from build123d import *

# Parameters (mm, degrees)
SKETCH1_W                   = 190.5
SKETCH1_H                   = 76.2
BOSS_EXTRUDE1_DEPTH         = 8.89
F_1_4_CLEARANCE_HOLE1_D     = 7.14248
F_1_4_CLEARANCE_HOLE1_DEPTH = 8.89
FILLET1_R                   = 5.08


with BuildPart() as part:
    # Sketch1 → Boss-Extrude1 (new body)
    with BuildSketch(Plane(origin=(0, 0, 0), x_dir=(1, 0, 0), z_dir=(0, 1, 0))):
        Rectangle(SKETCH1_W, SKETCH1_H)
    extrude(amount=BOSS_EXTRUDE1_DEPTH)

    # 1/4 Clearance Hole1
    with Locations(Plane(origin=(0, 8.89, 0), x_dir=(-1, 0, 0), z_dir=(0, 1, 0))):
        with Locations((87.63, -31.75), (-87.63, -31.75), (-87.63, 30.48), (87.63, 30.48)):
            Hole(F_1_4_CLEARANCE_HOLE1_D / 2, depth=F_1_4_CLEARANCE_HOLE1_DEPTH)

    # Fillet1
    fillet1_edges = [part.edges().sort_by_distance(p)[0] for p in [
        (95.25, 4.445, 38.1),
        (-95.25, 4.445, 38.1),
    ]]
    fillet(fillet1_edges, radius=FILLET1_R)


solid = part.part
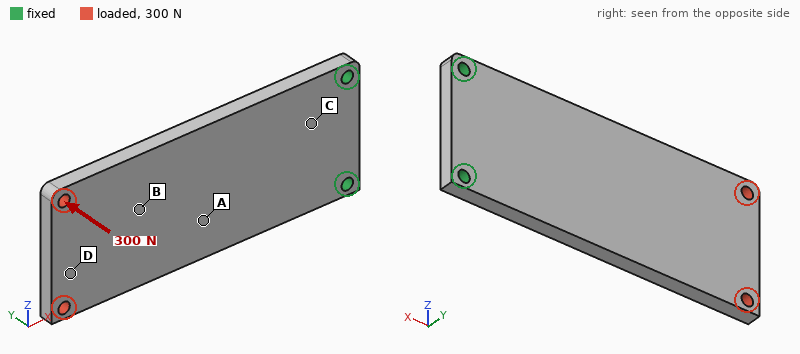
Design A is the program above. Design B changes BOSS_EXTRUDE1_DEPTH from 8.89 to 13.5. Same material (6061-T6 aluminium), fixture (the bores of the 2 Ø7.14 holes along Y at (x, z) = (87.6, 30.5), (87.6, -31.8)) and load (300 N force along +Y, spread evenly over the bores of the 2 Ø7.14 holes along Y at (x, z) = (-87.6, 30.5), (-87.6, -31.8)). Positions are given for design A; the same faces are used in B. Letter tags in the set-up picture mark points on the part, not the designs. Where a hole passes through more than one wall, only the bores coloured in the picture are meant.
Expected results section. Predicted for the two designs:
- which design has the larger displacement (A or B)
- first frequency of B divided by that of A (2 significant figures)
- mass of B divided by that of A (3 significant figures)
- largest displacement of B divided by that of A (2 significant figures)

A
1.5
1.52
0.30
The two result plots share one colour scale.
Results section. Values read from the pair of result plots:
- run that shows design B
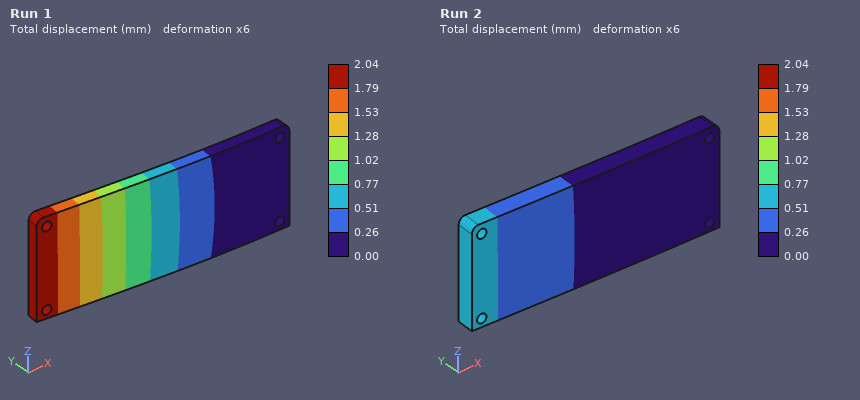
Run 2
